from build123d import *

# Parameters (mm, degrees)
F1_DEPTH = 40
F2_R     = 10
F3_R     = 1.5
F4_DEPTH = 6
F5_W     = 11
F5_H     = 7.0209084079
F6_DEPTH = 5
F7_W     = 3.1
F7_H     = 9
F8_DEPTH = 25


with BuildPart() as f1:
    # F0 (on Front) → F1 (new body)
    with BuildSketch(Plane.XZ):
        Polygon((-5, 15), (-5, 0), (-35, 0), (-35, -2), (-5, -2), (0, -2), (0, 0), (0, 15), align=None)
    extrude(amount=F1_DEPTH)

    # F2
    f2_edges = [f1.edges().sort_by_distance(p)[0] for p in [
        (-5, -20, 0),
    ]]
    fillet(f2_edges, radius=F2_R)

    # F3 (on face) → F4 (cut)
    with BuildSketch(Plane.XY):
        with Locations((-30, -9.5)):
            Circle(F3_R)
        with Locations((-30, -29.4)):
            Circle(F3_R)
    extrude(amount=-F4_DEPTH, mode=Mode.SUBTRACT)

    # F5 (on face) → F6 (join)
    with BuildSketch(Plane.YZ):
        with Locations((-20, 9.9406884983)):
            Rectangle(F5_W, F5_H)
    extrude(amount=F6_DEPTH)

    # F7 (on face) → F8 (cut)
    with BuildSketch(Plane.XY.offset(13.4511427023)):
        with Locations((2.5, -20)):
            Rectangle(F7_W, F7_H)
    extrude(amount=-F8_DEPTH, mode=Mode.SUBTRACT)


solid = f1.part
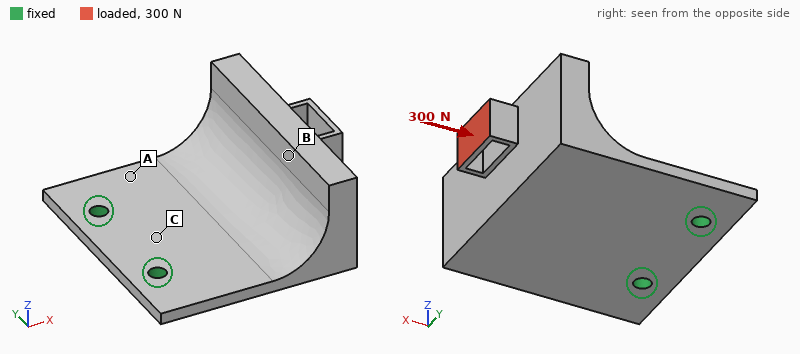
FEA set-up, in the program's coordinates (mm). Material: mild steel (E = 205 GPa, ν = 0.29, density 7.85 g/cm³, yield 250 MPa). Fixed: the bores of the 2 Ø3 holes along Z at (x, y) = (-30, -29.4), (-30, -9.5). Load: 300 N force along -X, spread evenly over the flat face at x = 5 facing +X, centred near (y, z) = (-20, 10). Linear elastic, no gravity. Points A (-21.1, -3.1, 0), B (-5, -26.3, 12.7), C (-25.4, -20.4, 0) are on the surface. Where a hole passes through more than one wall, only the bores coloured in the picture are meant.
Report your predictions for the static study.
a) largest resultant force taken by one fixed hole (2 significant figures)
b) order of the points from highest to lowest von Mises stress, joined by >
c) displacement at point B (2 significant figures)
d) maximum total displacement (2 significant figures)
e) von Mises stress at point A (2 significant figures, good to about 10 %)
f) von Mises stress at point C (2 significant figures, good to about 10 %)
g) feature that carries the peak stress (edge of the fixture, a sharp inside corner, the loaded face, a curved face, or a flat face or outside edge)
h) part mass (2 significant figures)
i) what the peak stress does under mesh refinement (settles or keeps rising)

160 N
A > C > B
0.23 mm
0.33 mm
120 MPa
100 MPa
edge of the fixture
54 g
keeps rising
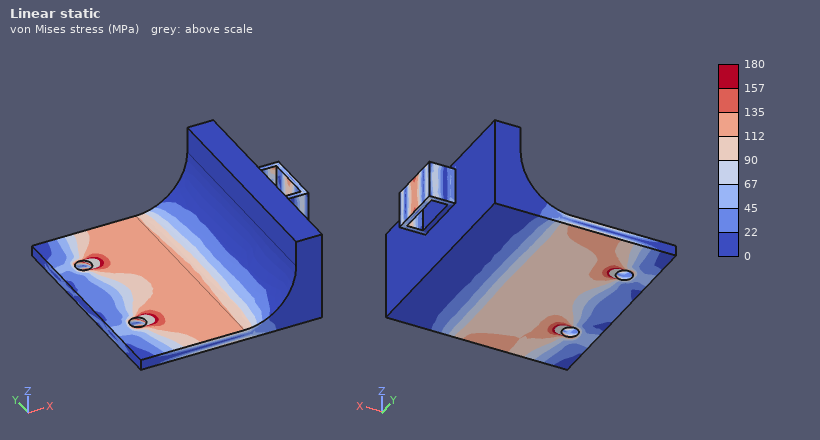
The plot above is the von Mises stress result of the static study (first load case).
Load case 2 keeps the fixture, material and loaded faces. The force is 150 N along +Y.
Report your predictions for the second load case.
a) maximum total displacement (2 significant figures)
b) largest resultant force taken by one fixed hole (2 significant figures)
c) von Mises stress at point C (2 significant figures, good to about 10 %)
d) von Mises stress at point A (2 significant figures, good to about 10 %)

32 µm
260 N
22 MPa
15 MPa
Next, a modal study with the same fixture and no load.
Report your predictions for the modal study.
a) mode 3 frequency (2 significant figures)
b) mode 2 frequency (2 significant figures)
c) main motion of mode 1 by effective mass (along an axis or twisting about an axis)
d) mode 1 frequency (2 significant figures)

4900 Hz
2000 Hz
along Z
700 Hz
